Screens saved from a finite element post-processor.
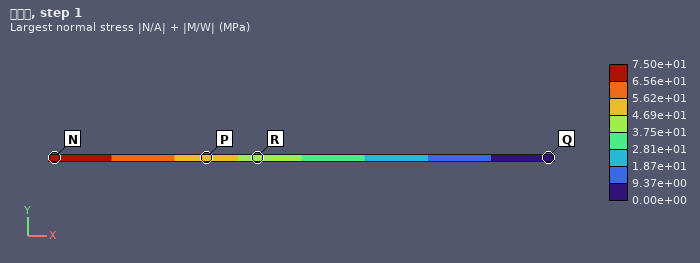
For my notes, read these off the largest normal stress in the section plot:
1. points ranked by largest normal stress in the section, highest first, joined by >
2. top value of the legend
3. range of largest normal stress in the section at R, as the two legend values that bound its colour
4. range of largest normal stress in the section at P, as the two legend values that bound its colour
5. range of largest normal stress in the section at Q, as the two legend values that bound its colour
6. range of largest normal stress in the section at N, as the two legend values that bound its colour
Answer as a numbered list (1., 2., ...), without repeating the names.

1. N > P > R > Q
2. 7.50e+01 MPa
3. 3.75e+01 to 4.69e+01 MPa
4. 4.69e+01 to 5.62e+01 MPa
5. 0.00e+00 to 9.37e+00 MPa
6. 6.56e+01 to 7.50e+01 MPa
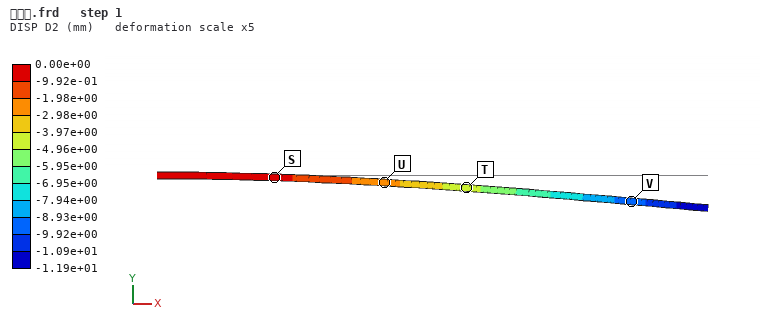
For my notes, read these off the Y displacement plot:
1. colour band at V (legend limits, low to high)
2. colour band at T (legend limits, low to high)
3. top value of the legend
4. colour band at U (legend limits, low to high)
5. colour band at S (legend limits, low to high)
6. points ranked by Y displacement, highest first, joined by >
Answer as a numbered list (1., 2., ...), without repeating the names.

1. -9.92e+00 to -8.93e+00 mm
2. -4.96e+00 to -3.97e+00 mm
3. 0.00e+00 mm
4. -2.98e+00 to -1.98e+00 mm
5. -9.92e-01 to 0.00e+00 mm
6. S > U > T > V
